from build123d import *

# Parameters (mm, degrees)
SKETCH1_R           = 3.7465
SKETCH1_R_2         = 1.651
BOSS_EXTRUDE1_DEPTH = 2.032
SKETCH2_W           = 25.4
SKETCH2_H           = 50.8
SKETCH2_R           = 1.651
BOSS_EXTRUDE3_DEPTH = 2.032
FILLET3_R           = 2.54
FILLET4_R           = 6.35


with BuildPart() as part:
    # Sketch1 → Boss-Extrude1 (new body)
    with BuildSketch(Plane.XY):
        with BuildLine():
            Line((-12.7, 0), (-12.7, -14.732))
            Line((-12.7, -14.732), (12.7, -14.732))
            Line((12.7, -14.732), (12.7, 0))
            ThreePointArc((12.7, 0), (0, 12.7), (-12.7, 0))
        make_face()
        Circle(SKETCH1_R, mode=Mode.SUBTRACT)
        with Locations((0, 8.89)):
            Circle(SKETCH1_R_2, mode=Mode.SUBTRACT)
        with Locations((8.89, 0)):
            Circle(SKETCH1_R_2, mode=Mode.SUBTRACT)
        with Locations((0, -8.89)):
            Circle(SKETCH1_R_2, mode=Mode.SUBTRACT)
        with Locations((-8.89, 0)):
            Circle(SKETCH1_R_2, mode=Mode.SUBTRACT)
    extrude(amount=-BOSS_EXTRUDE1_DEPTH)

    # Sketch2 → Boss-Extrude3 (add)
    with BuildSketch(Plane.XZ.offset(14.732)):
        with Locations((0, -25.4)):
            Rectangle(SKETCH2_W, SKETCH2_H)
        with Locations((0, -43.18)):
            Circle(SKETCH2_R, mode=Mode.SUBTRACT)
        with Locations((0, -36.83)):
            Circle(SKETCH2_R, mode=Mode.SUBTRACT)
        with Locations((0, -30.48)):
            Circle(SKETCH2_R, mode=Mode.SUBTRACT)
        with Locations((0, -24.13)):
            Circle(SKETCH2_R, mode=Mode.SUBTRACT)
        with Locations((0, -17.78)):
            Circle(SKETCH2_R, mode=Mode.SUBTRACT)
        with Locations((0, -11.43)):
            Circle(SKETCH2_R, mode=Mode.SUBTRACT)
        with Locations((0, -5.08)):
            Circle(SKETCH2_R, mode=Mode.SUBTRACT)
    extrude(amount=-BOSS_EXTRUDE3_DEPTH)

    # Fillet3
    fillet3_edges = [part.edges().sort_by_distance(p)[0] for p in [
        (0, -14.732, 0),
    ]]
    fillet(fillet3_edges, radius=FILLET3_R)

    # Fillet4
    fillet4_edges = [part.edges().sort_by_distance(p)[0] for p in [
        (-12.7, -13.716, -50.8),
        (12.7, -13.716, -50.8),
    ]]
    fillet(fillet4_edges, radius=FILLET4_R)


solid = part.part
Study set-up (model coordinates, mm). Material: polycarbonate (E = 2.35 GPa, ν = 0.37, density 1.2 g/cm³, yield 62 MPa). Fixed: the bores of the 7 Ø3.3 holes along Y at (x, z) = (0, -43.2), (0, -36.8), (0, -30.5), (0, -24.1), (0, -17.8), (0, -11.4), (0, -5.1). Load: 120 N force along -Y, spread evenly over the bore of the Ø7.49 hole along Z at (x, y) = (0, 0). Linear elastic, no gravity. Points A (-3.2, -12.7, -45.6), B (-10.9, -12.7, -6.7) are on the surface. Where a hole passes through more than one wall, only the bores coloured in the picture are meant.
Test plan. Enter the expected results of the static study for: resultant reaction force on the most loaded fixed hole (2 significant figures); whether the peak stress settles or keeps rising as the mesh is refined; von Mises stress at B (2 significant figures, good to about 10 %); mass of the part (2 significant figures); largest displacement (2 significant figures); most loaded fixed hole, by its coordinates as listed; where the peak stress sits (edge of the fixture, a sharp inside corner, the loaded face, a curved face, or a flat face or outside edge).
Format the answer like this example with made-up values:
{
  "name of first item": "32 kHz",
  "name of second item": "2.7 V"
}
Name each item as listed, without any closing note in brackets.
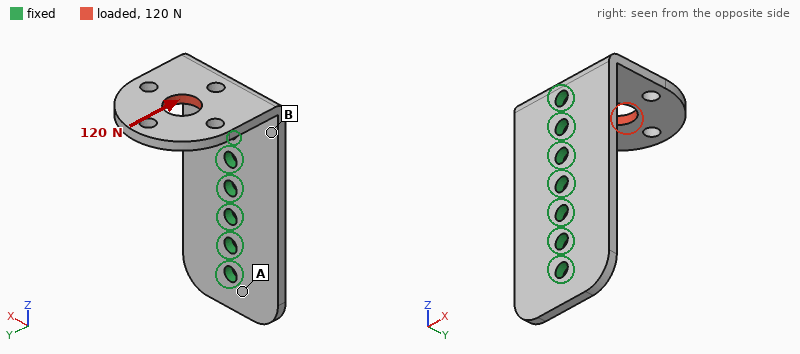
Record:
{
  "resultant reaction force on the most loaded fixed hole": "130 N",
  "whether the peak stress settles or keeps rising as the mesh is refined": "keeps rising",
  "von Mises stress at B": "4.7 MPa",
  "mass of the part": "4.1 g",
  "largest displacement": "0.68 mm",
  "most loaded fixed hole, by its coordinates as listed": "(0, -5.1)",
  "where the peak stress sits": "edge of the fixture"
}
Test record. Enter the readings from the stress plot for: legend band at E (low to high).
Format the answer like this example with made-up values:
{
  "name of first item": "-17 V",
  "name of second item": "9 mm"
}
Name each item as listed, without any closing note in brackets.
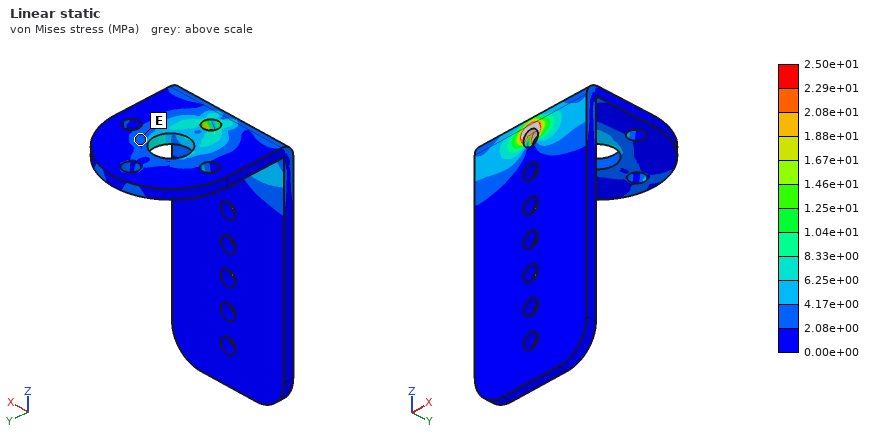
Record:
{
  "legend band at E": "2.08e+00 to 4.17e+00 MPa"
}
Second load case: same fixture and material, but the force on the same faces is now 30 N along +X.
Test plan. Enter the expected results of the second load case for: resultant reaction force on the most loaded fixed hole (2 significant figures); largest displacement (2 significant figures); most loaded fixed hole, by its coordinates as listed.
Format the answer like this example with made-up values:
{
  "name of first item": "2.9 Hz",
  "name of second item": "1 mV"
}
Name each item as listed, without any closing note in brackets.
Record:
{
  "resultant reaction force on the most loaded fixed hole": "30 N",
  "largest displacement": "0.66 mm",
  "most loaded fixed hole, by its coordinates as listed": "(0, -5.1)"
}
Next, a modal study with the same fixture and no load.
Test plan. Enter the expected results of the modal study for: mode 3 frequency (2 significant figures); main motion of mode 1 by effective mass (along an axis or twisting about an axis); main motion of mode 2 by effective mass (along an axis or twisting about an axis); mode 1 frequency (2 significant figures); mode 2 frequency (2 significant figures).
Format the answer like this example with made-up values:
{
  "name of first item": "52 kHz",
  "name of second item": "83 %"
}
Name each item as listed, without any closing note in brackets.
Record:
{
  "mode 3 frequency": "1800 Hz",
  "main motion of mode 1 by effective mass": "along Z",
  "main motion of mode 2 by effective mass": "along X",
  "mode 1 frequency": "640 Hz",
  "mode 2 frequency": "1100 Hz"
}
